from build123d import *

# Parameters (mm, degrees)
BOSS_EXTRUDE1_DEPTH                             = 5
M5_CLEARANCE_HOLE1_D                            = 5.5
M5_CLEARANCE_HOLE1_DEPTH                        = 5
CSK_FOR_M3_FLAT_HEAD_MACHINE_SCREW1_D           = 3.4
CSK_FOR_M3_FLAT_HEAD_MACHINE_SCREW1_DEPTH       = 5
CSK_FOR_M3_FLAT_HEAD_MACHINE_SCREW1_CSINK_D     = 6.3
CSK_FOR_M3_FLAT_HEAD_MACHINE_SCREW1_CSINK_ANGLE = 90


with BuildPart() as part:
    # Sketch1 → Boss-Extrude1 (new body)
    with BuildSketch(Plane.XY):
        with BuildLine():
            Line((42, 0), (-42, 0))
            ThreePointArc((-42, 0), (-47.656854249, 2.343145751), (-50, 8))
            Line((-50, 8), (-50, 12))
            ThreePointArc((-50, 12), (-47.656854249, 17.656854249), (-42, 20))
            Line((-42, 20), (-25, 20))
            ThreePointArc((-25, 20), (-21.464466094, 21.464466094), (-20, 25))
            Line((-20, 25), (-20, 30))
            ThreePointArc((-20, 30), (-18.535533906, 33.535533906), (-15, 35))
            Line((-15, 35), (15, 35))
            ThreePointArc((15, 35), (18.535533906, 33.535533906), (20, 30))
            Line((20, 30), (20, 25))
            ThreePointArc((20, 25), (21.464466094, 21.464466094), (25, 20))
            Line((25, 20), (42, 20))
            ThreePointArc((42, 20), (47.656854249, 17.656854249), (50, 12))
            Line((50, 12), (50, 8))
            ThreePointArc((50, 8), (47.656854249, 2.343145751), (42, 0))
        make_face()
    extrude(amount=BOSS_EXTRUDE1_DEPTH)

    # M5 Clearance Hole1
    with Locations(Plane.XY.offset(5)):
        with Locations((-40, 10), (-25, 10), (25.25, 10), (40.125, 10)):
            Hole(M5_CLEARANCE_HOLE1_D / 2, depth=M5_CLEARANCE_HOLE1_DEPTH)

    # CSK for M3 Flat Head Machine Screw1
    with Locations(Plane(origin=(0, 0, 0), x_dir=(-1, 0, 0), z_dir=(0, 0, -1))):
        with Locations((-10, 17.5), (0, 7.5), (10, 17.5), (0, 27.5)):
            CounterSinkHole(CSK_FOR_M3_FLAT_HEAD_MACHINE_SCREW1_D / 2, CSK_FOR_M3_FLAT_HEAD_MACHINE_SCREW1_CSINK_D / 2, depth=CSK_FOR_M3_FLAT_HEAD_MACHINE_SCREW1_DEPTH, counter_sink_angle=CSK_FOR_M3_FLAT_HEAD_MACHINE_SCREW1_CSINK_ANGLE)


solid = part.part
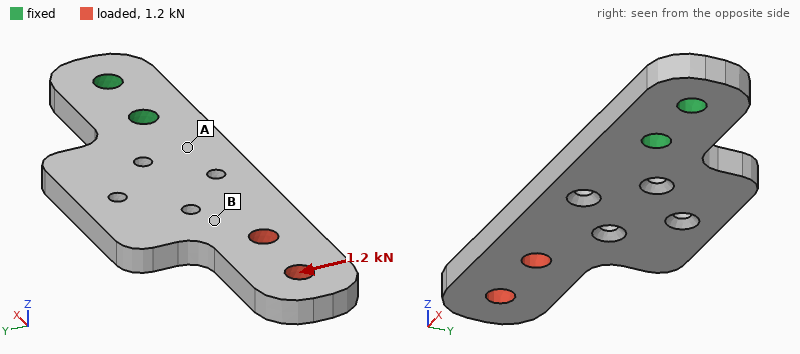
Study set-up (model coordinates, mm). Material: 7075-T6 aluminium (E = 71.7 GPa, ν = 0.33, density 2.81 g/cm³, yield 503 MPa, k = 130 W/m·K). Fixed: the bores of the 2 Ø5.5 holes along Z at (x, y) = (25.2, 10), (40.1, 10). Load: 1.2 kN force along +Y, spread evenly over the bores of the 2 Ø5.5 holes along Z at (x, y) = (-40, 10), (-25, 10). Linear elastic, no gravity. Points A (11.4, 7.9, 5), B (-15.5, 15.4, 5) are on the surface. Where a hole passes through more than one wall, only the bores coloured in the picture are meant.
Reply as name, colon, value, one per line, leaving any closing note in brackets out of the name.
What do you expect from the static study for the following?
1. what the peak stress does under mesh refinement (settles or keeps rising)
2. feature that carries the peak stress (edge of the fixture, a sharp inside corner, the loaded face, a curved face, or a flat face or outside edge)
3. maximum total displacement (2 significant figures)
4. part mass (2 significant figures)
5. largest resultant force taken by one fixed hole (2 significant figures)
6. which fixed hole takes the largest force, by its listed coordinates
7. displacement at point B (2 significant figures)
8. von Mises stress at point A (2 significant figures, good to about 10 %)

what the peak stress does under mesh refinement: keeps rising
feature that carries the peak stress: edge of the fixture
maximum total displacement: 0.46 mm
part mass: 34 g
largest resultant force taken by one fixed hole: 3.7 kN
which fixed hole takes the largest force, by its listed coordinates: (25.2, 10)
displacement at point B: 0.22 mm
von Mises stress at point A: 57 MPa
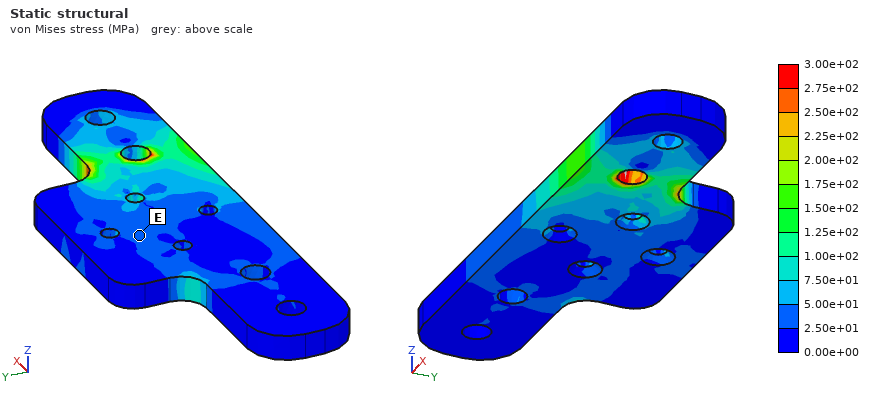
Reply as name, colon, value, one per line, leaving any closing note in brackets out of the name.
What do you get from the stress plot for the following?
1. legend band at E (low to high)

legend band at E: 2.50e+01 to 5.00e+01 MPa
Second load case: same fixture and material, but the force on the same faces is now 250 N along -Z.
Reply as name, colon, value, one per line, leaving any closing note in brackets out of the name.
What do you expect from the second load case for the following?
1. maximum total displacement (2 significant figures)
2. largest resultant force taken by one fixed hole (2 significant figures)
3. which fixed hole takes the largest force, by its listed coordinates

maximum total displacement: 1.2 mm
largest resultant force taken by one fixed hole: 440 N
which fixed hole takes the largest force, by its listed coordinates: (25.2, 10)
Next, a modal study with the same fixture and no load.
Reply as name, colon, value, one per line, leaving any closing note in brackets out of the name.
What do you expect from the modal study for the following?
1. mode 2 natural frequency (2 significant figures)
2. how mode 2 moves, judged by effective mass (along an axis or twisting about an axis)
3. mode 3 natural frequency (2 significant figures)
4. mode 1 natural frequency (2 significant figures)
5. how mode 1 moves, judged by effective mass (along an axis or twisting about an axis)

mode 2 natural frequency: 2700 Hz
how mode 2 moves, judged by effective mass: along Y
mode 3 natural frequency: 2900 Hz
mode 1 natural frequency: 830 Hz
how mode 1 moves, judged by effective mass: along Z
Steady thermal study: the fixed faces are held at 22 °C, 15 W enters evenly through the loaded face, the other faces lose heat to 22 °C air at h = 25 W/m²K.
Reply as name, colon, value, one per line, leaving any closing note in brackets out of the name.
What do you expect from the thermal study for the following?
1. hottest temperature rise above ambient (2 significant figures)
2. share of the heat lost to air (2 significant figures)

hottest temperature rise above ambient: 50 K
share of the heat lost to air: 22 %
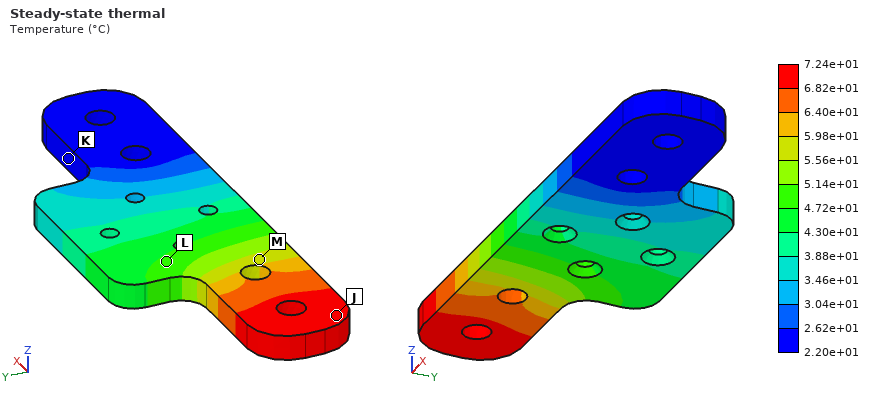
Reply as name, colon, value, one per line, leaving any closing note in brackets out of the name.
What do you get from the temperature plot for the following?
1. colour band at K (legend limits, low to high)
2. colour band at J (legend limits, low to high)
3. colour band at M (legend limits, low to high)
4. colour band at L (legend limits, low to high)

colour band at K: 2.20e+01 to 2.62e+01 °C
colour band at J: 6.82e+01 to 7.24e+01 °C
colour band at M: 5.56e+01 to 5.98e+01 °C
colour band at L: 4.72e+01 to 5.14e+01 °C
